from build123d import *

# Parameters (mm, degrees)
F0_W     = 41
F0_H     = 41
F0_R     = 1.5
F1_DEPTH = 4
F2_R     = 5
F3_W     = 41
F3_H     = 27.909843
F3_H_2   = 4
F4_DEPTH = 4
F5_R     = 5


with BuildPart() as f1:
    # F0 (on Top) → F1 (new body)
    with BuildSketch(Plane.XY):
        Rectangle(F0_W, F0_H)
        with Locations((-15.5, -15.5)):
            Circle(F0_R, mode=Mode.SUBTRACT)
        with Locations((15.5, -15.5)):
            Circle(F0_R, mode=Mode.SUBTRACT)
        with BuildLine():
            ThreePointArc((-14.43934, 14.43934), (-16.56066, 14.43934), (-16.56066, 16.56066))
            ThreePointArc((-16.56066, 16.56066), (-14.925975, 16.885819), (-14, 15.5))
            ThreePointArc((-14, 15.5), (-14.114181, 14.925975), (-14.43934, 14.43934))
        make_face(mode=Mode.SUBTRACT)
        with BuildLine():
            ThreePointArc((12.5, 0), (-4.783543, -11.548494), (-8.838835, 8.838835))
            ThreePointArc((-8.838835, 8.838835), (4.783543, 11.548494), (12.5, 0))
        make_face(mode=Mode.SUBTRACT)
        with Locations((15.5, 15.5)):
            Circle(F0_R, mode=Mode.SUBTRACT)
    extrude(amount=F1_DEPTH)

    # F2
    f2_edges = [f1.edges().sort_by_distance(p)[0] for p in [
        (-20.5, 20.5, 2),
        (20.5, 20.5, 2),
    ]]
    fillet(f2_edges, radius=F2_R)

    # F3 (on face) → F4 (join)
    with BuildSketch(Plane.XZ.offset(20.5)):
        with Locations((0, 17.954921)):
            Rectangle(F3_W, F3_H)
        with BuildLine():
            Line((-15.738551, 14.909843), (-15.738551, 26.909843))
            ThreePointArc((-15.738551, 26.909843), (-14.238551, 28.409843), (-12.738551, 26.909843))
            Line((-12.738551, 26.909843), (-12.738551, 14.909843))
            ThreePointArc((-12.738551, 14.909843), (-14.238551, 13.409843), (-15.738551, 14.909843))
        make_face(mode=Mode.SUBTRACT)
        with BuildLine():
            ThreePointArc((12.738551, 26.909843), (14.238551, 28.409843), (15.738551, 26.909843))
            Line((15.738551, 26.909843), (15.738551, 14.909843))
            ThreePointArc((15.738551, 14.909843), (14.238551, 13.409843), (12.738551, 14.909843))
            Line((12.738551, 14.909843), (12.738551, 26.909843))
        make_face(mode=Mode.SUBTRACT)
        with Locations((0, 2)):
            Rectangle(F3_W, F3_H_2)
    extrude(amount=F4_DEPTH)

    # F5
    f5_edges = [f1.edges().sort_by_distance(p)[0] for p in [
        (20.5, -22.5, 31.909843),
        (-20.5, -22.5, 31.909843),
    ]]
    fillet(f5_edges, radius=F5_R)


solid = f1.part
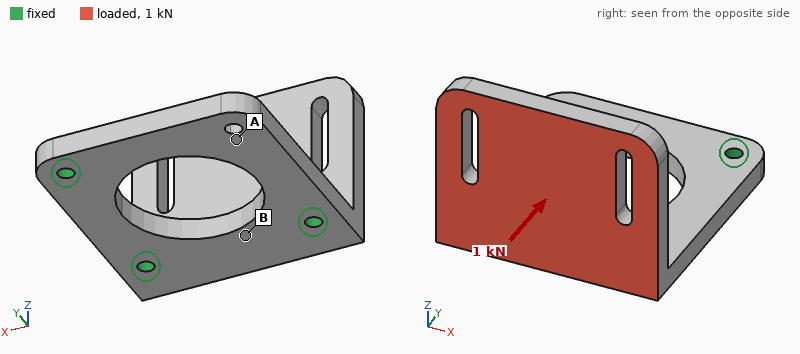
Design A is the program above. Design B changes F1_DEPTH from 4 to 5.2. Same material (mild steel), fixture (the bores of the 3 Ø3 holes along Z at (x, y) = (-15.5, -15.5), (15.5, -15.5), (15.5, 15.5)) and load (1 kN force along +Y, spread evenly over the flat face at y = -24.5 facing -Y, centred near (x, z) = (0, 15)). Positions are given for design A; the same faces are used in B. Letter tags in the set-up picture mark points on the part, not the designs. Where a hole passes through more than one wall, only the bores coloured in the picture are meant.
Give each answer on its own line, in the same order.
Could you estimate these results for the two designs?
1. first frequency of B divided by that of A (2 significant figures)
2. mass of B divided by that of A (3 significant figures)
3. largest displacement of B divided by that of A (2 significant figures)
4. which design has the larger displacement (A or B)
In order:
1.2
1.15
0.65
A
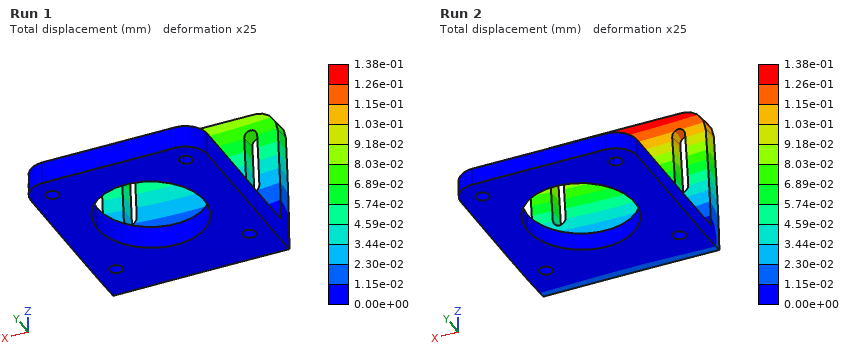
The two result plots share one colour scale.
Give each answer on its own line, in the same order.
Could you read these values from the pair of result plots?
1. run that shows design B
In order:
Run 1
